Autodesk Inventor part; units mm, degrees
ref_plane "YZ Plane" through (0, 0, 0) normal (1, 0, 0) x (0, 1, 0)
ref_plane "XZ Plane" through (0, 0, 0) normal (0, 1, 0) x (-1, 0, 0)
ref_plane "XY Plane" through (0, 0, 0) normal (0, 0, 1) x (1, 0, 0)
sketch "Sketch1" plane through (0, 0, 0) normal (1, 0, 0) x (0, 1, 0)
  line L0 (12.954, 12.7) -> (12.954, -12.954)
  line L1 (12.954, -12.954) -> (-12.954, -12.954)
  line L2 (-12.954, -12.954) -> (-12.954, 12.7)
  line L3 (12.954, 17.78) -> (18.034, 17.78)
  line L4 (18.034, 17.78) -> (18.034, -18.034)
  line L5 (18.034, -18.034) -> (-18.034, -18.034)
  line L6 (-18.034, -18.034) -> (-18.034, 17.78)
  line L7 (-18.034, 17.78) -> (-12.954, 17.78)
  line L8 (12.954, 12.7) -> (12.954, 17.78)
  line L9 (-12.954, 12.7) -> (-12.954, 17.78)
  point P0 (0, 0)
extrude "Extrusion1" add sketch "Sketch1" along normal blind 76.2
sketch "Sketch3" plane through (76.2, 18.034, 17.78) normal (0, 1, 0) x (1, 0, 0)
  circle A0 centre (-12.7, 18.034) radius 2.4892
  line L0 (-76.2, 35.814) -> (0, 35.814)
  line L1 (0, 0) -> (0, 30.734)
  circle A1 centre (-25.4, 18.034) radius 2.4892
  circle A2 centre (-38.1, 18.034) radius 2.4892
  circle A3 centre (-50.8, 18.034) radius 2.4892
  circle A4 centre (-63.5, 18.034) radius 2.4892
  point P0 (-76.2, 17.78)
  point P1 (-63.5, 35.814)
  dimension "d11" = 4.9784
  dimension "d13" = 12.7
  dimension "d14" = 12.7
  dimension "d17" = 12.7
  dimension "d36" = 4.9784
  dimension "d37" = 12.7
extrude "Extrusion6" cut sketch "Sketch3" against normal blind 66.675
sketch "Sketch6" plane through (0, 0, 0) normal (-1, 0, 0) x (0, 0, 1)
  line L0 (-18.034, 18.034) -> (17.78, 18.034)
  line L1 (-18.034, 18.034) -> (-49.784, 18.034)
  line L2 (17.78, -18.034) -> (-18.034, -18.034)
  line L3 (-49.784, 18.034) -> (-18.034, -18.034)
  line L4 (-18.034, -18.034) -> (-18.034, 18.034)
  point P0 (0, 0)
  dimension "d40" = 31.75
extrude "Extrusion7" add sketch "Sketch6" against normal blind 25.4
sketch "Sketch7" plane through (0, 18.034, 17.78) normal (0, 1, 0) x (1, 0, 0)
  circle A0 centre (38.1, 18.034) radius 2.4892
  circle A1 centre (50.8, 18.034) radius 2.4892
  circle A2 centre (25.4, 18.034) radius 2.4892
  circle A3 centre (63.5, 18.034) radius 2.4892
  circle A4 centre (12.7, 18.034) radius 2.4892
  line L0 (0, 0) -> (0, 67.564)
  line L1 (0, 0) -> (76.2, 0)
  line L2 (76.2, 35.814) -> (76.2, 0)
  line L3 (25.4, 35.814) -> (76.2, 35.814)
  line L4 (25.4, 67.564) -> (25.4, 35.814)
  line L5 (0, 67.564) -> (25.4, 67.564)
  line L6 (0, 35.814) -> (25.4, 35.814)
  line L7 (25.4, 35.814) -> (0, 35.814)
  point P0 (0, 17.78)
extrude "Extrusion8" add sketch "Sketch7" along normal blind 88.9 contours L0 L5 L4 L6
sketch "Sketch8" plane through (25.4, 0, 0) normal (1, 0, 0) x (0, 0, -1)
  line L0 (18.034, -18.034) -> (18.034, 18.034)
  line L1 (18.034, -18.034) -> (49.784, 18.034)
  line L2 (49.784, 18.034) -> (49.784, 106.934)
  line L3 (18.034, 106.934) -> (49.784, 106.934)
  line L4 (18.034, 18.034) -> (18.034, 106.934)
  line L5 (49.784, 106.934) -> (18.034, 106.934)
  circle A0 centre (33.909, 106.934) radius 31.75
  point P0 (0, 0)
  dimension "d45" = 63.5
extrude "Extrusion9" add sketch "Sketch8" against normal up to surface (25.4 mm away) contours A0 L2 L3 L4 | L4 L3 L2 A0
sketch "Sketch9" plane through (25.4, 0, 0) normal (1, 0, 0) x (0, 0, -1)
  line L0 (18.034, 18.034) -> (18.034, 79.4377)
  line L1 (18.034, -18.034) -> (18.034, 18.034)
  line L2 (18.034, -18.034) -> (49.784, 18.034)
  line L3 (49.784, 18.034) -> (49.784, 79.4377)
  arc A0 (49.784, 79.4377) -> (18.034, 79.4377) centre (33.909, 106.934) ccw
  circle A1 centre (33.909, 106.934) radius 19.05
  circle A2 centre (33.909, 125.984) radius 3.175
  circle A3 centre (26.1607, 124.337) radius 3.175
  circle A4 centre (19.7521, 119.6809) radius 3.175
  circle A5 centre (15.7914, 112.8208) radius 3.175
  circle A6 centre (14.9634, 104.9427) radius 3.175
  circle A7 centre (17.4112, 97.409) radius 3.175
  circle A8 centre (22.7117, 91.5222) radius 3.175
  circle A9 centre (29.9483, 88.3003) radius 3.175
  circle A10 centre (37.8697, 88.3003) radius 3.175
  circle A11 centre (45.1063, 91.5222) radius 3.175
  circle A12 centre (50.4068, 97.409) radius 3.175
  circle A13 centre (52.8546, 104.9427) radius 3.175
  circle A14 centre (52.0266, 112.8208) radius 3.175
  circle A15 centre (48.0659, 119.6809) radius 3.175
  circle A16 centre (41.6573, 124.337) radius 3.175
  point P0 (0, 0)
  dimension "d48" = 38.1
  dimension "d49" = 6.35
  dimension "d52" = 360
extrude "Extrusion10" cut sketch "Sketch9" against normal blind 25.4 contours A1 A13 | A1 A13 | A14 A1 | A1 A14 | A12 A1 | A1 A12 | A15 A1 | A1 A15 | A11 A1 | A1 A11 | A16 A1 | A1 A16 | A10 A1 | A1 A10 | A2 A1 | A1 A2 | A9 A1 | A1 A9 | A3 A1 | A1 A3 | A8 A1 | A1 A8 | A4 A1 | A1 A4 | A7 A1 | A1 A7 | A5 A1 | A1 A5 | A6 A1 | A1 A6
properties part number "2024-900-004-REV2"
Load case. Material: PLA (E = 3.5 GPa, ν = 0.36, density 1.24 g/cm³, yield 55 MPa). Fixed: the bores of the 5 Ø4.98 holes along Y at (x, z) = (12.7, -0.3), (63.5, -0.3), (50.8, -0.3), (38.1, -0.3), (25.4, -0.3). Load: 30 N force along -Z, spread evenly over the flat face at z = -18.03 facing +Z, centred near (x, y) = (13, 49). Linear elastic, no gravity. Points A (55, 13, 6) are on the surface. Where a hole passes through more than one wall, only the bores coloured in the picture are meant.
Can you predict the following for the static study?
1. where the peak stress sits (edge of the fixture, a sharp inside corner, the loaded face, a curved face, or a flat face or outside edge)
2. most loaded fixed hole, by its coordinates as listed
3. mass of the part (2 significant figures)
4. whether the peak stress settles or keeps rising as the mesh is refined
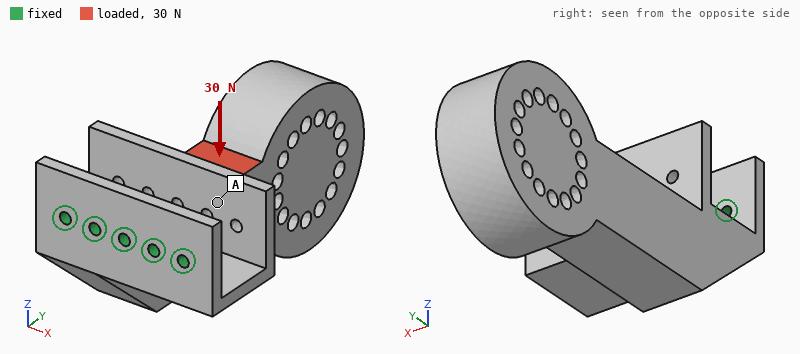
edge of the fixture
(12.7, -0.3)
210 g
keeps rising
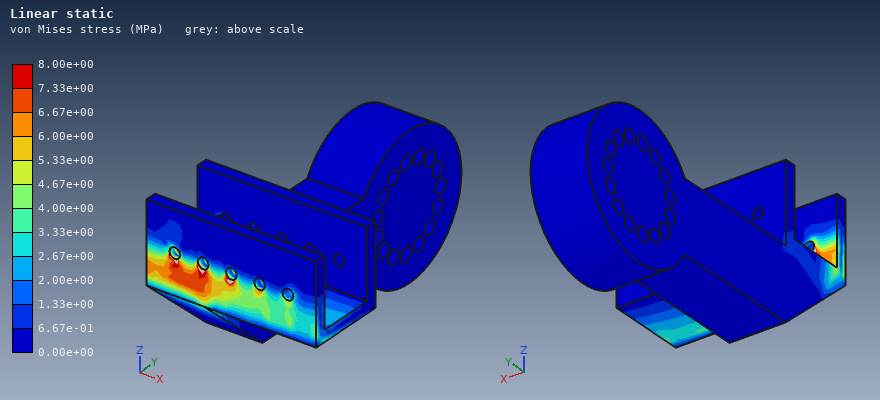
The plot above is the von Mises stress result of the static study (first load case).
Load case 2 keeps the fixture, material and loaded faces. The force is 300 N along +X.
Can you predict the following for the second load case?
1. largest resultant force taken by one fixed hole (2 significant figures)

330 N
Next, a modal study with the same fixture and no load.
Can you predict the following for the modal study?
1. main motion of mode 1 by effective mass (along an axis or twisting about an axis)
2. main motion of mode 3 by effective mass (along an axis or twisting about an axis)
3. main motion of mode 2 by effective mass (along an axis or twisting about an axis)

along Z
twisting about Y
along X
